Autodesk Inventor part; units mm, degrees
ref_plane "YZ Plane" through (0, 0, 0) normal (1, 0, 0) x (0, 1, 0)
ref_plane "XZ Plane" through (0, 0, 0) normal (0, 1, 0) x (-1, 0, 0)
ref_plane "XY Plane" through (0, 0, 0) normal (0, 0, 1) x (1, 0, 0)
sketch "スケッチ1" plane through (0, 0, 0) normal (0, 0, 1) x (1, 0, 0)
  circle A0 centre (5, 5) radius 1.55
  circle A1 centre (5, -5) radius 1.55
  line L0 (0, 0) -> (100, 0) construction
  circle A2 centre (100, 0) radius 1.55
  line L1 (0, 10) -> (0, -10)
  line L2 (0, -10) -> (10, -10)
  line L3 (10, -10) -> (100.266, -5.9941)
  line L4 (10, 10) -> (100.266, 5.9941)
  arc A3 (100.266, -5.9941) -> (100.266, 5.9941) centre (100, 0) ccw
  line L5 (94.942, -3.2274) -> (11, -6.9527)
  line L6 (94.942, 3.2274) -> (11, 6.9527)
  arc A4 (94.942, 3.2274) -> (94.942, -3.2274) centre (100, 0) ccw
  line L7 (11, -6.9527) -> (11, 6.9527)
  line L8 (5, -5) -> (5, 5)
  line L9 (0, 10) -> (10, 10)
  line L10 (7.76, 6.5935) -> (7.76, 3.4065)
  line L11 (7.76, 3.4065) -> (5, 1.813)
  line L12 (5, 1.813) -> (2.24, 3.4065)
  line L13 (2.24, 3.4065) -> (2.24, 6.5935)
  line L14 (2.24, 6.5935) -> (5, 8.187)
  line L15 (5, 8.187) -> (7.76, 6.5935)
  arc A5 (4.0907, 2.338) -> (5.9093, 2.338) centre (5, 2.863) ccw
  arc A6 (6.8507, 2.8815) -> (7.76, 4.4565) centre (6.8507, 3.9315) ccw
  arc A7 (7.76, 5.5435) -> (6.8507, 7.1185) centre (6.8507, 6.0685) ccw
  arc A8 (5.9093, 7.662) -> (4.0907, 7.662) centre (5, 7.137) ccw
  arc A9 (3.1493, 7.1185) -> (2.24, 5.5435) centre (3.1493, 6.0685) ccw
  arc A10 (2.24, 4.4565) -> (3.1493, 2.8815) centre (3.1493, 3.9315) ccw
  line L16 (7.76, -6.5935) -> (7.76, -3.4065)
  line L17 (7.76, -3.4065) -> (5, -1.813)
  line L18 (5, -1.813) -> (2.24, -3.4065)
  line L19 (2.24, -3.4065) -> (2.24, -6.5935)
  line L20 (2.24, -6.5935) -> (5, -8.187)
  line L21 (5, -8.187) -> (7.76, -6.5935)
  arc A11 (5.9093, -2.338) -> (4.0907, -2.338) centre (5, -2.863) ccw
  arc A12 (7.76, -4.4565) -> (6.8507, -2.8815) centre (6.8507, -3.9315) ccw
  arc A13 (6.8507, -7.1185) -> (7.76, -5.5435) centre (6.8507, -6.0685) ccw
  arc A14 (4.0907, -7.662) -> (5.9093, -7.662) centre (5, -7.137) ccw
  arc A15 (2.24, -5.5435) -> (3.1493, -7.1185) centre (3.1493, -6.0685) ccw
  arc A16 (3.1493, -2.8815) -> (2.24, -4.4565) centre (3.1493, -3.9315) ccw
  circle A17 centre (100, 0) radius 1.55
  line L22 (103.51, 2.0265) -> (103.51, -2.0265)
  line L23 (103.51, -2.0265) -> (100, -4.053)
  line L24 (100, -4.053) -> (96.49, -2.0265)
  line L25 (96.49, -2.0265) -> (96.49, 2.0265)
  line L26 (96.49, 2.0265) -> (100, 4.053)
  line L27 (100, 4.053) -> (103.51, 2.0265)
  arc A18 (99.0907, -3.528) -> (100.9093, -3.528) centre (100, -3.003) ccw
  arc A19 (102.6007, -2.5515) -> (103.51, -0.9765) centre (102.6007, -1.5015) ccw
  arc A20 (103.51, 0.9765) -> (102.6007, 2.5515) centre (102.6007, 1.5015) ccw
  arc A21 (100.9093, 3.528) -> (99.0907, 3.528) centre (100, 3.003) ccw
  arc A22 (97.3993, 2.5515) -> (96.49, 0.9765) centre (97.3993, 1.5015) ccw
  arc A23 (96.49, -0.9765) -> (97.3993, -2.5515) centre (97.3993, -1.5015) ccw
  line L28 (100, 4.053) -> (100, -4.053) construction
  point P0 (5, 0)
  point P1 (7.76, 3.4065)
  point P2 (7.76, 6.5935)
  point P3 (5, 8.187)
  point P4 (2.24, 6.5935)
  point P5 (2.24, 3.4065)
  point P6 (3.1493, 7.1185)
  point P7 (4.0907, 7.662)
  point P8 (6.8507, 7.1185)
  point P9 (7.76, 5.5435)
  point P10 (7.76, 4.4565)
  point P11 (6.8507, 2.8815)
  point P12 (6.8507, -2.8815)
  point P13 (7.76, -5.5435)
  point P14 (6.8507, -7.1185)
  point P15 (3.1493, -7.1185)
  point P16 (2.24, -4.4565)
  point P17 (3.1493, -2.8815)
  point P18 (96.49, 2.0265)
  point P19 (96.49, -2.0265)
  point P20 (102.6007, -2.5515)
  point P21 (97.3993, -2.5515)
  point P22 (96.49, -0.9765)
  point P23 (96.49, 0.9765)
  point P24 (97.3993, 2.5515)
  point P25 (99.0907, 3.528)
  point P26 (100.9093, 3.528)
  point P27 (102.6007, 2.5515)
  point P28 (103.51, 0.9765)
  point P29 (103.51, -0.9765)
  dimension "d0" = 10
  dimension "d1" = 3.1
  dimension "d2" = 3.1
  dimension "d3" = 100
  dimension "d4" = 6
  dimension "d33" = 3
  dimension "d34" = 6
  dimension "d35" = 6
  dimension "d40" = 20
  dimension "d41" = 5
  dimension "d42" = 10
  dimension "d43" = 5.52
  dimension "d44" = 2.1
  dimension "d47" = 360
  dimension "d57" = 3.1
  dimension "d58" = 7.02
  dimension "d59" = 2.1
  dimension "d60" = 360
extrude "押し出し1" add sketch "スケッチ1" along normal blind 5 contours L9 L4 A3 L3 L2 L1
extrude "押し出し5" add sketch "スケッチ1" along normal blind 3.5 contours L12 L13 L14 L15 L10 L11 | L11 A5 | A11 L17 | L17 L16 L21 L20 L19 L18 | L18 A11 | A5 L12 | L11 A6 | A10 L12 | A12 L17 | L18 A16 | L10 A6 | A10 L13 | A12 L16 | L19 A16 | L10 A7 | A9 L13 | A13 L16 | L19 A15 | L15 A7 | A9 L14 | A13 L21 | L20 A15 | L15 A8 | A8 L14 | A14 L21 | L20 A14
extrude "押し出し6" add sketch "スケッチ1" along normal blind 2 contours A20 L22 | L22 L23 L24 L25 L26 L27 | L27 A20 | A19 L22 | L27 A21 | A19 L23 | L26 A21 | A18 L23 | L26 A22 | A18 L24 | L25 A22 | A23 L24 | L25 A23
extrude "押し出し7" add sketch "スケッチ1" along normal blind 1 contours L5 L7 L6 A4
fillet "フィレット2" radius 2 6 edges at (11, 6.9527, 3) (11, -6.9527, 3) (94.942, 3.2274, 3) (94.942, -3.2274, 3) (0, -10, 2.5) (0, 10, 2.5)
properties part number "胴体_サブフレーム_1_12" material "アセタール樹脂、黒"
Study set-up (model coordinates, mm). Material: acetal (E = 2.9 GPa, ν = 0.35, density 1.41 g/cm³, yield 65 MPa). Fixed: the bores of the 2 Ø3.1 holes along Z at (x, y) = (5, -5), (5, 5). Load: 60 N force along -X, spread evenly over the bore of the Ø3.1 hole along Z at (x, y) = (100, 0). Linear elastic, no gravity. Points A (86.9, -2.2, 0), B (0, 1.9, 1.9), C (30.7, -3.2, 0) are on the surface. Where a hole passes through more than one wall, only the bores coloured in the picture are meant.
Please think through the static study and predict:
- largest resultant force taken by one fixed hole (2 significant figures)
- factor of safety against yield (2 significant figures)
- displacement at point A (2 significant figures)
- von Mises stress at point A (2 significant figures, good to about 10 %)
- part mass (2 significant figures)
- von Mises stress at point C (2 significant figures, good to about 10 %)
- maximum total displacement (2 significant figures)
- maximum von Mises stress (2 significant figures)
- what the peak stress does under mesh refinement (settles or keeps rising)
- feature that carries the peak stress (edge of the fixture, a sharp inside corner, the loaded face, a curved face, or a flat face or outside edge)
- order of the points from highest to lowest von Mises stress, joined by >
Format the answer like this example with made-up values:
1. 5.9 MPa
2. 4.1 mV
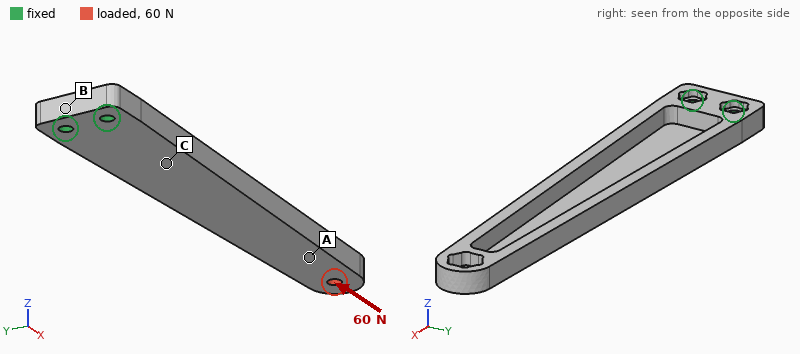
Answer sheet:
1. 30 N
2. 10
3. 0.64 mm
4. 3.4 MPa
5. 6.8 g
6. 2.5 MPa
7. 1.0 mm
8. 6.4 MPa
9. settles
10. the loaded face
11. A > C > B
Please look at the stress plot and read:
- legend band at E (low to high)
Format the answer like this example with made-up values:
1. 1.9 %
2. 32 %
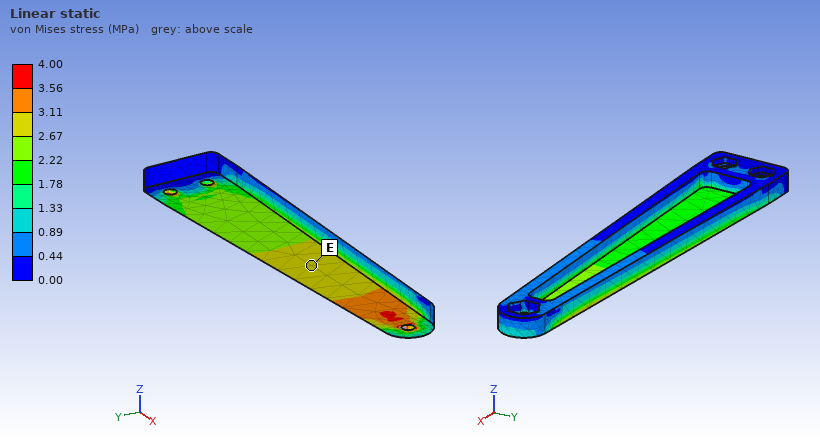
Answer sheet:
1. 2.67 to 3.11 MPa
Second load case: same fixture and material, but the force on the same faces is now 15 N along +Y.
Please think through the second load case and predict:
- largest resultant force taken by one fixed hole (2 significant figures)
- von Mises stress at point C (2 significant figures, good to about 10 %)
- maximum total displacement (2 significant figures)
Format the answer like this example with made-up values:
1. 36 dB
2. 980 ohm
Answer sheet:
1. 120 N
2. 2.0 MPa
3. 1.0 mm
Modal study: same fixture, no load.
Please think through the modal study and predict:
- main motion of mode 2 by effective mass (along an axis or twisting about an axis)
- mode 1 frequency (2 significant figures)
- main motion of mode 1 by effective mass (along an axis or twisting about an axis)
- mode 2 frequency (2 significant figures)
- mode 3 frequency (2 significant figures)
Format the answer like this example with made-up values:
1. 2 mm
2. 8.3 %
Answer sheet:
1. along Y
2. 130 Hz
3. along Z
4. 460 Hz
5. 710 Hz
